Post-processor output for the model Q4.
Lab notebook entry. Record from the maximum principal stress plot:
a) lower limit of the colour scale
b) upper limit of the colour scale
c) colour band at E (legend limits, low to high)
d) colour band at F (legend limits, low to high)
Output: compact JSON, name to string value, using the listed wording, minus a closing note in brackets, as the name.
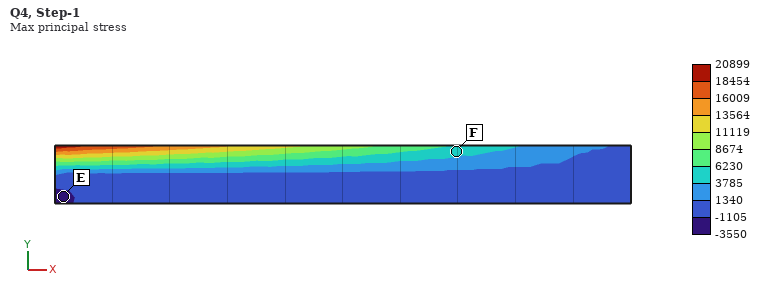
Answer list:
{"lower limit of the colour scale": "-3550", "upper limit of the colour scale": "20899", "colour band at E": "-3550 to -1105", "colour band at F": "3785 to 6230"}
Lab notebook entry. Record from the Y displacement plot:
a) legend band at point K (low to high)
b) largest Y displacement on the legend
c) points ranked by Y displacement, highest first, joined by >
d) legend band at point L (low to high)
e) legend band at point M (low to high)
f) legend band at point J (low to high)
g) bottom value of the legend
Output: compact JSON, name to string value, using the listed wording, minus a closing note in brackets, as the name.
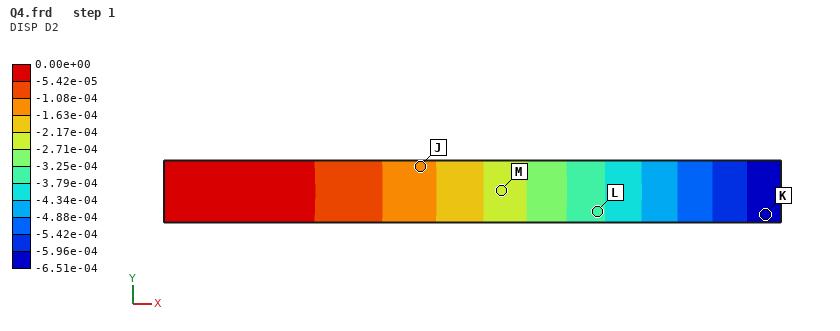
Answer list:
{"legend band at point K": "-6.51e-04 to -5.96e-04", "largest Y displacement on the legend": "0.00e+00", "points ranked by Y displacement, highest first, joined by >": "J > M > L > K", "legend band at point L": "-3.79e-04 to -3.25e-04", "legend band at point M": "-2.71e-04 to -2.17e-04", "legend band at point J": "-1.63e-04 to -1.08e-04", "bottom value of the legend": "-6.51e-04"}
